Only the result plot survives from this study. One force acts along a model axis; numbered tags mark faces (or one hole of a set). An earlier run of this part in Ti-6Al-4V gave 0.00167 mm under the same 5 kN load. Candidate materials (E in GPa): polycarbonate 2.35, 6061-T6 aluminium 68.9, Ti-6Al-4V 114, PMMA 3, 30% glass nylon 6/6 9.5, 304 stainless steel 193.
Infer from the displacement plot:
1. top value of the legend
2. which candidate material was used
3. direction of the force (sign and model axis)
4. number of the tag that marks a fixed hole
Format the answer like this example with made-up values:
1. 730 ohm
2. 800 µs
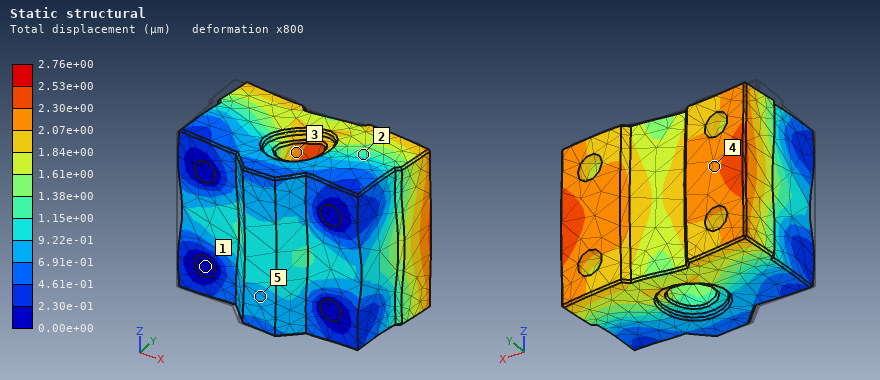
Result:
1. 2.76e+00 µm
2. 6061-T6 aluminium
3. +X
4. 1
